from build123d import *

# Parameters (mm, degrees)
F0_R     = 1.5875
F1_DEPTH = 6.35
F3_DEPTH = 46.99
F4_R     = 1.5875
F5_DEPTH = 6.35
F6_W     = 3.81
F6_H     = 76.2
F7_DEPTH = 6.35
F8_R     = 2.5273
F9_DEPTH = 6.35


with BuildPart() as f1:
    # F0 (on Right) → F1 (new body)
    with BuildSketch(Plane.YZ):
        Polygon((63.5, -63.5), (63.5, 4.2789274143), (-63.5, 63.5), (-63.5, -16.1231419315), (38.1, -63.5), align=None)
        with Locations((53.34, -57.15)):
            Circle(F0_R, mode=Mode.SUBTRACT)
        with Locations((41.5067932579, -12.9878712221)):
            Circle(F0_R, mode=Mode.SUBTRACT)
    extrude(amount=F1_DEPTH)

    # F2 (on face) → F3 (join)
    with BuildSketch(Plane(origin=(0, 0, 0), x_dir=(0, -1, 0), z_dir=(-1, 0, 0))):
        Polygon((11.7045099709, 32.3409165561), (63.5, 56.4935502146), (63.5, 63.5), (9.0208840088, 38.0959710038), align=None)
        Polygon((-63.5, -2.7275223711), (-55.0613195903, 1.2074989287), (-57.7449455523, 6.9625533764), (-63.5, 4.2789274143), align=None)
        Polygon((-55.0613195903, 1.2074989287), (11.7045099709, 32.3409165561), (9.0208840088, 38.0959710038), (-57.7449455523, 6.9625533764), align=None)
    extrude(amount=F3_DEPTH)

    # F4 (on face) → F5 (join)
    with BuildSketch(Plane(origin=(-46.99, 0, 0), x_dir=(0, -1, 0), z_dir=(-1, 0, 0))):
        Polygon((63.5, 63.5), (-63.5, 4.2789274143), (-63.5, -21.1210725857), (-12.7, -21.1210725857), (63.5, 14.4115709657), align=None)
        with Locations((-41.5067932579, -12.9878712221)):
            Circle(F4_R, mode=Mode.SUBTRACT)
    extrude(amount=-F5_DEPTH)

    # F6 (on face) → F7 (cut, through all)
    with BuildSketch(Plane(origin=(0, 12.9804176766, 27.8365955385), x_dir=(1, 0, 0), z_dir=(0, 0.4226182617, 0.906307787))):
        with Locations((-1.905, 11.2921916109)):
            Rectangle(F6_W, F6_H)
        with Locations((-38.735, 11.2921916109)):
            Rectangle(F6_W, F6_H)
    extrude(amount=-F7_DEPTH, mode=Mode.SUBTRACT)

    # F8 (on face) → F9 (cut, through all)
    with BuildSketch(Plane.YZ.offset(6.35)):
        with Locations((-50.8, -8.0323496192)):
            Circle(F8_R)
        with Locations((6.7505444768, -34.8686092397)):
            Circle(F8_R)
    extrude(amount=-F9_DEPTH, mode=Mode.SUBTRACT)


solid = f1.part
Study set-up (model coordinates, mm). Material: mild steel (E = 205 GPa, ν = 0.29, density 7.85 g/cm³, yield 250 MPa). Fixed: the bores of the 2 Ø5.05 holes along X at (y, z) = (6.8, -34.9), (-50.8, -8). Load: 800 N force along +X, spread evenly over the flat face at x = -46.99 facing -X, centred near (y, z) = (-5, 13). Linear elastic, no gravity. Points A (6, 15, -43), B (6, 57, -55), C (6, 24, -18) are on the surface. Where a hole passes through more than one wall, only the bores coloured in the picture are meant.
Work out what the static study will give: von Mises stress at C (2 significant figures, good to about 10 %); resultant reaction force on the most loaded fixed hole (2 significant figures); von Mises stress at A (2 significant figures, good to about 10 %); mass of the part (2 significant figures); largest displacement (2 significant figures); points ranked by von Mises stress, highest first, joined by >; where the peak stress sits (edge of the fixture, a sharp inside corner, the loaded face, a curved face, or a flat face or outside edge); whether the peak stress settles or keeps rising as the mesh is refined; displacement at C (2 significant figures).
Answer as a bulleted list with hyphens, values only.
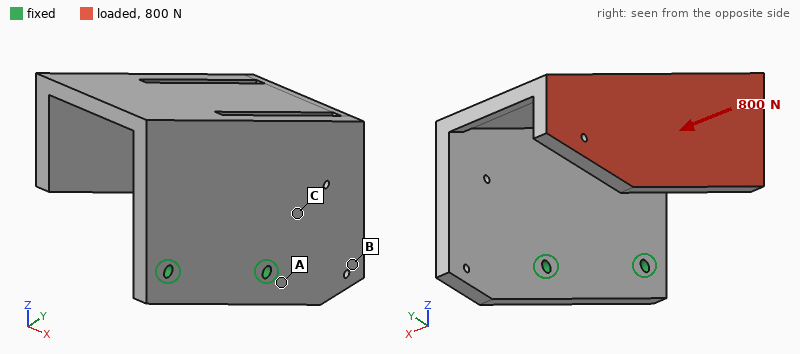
- 15 MPa
- 420 N
- 25 MPa
- 1.0 kg
- 0.15 mm
- A > C > B
- edge of the fixture
- keeps rising
- 0.024 mm
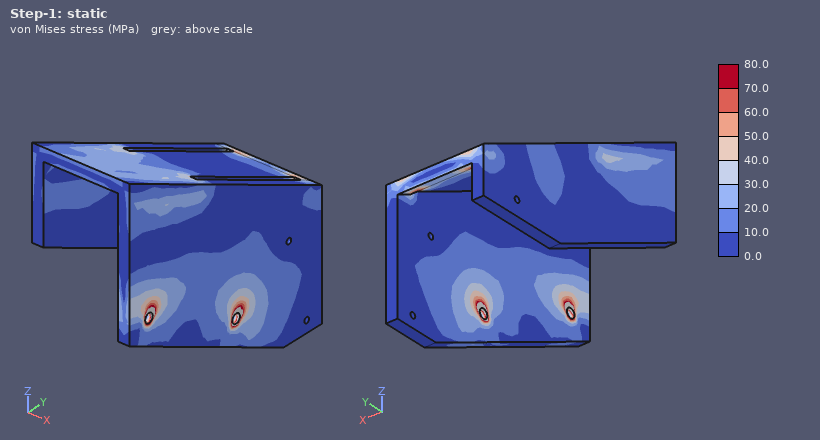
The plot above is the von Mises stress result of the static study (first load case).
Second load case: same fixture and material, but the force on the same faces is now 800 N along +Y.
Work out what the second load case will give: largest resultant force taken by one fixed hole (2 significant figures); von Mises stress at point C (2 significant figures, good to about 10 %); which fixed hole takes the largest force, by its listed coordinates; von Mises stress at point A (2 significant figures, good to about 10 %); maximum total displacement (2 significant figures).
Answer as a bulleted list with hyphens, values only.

- 820 N
- 25 MPa
- (-50.8, -8)
- 39 MPa
- 0.25 mm
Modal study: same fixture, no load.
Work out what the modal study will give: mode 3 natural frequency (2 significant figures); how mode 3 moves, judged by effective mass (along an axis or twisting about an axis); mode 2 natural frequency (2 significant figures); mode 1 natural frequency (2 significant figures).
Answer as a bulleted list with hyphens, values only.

- 680 Hz
- along X
- 570 Hz
- 370 Hz
